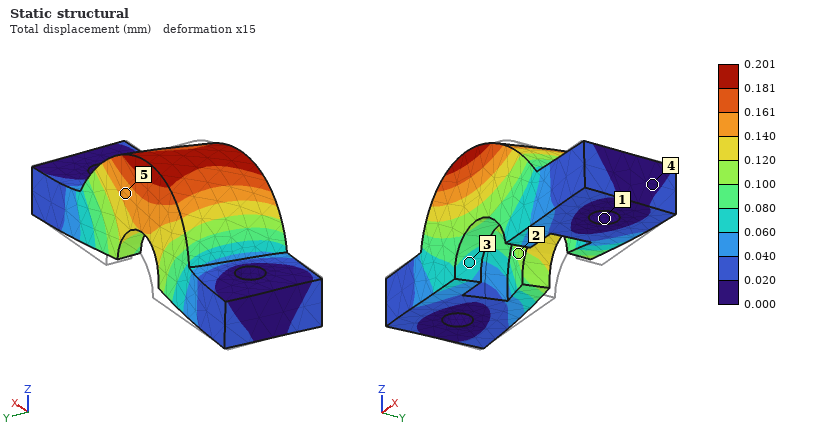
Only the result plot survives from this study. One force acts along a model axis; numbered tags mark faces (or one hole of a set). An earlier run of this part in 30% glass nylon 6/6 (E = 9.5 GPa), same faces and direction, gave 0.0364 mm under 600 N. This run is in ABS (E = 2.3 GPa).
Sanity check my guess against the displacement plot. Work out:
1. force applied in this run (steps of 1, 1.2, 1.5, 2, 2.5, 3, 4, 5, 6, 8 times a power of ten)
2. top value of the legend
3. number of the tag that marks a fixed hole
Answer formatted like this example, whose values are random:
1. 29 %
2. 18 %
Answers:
1. 800 N
2. 0.201 mm
3. 1
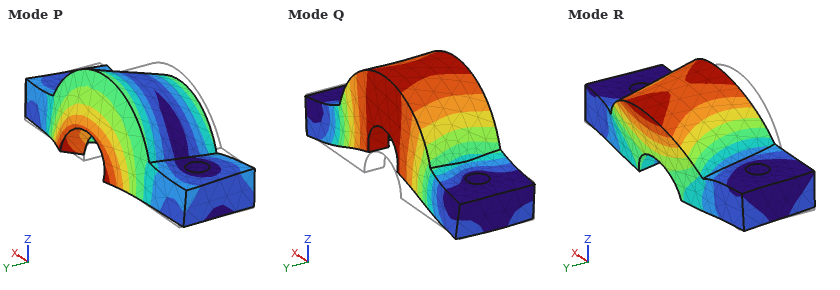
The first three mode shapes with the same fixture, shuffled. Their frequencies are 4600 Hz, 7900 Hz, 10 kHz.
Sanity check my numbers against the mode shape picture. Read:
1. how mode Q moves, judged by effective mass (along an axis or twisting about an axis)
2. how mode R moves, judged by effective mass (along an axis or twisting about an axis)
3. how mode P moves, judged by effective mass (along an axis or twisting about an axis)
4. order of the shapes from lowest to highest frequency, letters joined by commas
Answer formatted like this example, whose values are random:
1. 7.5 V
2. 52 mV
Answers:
1. along Z
2. along Y
3. along Y
4. R, Q, P
